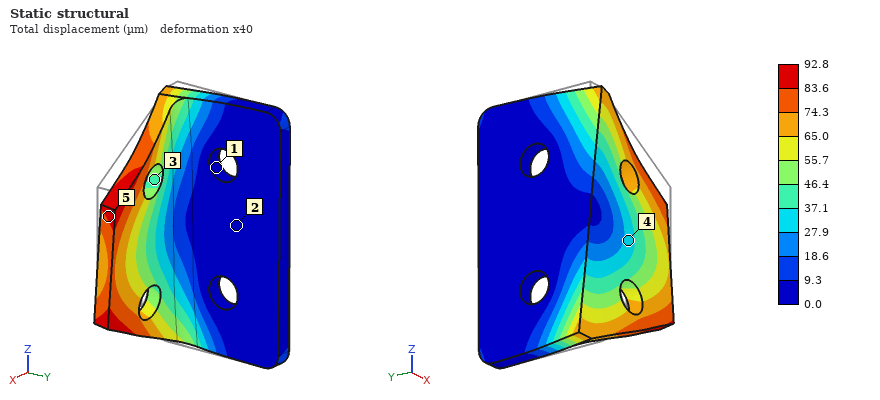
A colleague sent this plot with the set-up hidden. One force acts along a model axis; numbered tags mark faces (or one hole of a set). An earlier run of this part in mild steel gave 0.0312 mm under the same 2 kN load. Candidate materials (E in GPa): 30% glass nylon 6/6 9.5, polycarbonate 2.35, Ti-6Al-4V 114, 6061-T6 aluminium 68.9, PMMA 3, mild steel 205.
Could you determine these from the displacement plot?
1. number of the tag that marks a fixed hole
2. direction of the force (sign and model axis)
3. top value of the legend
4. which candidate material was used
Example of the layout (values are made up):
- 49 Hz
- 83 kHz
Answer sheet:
- 1
- -Z
- 92.8 µm
- 6061-T6 aluminium
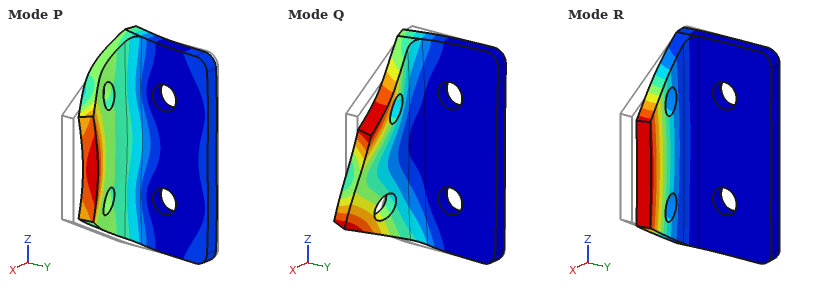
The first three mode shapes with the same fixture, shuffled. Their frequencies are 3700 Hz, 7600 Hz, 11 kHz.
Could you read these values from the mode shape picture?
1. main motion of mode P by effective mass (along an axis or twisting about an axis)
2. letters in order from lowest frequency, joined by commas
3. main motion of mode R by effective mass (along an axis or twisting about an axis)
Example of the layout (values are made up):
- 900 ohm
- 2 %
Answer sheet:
- along X
- R, Q, P
- along Y
